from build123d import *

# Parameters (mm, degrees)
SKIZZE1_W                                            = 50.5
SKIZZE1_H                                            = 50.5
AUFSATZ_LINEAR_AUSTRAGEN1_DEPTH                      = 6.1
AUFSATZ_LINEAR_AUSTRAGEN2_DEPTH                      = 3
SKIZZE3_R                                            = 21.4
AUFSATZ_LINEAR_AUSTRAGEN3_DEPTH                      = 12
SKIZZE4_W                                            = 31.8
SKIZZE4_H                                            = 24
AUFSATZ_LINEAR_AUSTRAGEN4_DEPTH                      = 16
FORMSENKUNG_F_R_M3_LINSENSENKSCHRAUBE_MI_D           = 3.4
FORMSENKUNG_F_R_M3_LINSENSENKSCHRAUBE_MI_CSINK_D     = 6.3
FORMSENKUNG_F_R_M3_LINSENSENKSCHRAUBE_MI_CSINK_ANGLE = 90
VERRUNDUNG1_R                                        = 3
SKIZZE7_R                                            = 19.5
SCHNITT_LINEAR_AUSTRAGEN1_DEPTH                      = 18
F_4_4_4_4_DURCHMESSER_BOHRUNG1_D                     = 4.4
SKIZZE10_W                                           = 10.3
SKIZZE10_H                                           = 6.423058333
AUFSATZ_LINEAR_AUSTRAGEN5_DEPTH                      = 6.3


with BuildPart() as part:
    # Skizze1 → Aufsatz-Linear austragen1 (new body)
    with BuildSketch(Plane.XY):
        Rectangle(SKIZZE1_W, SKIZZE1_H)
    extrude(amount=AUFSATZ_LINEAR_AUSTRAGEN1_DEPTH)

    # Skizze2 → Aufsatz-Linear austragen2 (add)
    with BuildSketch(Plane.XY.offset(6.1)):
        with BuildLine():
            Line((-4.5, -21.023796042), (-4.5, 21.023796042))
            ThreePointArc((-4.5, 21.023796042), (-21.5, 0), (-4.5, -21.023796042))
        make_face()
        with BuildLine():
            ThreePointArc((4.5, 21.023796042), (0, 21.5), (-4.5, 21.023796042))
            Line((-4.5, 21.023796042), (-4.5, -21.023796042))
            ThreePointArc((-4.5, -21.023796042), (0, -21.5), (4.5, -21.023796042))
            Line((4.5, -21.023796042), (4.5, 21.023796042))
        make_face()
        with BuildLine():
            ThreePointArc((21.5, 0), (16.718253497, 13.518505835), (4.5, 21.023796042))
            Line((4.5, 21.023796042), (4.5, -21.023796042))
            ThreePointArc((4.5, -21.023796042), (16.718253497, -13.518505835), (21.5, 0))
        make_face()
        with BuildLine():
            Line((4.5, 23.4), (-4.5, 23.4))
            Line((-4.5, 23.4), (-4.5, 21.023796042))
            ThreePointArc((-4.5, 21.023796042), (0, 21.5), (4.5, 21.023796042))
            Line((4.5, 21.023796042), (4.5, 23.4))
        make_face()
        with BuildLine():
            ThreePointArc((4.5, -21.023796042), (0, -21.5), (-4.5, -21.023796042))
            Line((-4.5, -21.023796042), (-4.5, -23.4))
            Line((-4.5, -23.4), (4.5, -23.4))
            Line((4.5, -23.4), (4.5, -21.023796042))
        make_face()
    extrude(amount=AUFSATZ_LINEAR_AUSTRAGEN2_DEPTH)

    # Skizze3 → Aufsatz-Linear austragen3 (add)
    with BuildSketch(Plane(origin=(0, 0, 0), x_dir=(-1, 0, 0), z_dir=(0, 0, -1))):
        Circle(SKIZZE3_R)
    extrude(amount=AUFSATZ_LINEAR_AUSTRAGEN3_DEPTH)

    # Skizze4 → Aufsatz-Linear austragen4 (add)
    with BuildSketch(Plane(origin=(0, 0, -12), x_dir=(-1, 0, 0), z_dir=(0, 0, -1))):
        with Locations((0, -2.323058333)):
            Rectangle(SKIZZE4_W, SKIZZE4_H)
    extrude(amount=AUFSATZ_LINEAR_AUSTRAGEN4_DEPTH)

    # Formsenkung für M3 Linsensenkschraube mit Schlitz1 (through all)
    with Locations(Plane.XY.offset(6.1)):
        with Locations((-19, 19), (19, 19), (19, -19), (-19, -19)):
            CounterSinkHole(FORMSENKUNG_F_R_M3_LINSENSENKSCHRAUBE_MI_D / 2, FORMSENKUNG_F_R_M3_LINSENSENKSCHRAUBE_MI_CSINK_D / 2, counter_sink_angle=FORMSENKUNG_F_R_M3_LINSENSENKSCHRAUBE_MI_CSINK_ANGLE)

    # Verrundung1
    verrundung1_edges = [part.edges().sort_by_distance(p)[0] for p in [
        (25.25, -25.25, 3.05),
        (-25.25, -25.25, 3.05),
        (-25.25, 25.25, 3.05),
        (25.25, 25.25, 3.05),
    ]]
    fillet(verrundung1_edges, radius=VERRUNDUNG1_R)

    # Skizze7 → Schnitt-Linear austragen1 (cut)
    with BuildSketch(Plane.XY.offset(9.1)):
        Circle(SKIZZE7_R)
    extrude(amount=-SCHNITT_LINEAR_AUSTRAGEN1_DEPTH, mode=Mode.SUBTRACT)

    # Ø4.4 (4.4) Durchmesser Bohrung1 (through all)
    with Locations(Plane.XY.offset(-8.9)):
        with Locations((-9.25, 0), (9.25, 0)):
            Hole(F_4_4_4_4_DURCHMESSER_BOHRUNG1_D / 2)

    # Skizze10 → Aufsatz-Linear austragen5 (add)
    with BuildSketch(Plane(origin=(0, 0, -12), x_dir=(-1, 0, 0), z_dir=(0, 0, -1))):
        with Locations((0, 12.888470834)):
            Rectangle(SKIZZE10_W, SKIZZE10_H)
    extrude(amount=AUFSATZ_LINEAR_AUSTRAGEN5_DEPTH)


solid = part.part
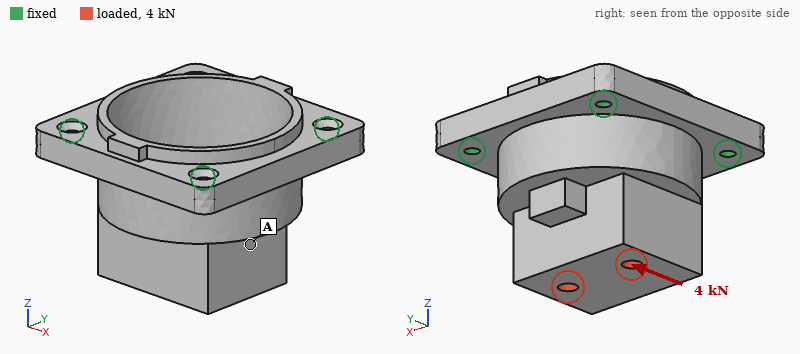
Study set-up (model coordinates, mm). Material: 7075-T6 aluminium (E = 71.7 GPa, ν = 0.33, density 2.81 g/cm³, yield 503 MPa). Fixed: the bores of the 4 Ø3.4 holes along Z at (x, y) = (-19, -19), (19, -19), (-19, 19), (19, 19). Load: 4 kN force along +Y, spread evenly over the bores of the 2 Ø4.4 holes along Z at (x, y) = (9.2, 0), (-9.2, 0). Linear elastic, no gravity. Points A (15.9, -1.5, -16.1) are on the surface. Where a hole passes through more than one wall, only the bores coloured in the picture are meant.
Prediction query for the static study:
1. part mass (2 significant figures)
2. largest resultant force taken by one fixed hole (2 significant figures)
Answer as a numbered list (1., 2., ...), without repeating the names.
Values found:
1. 77 g
2. 1.6 kN
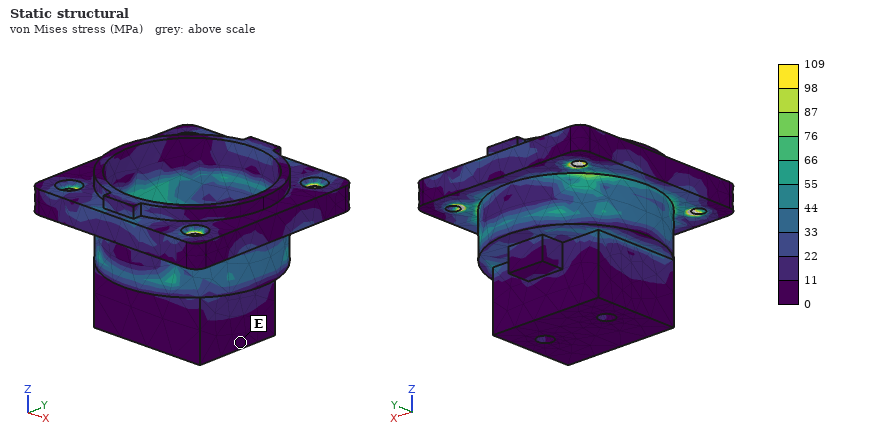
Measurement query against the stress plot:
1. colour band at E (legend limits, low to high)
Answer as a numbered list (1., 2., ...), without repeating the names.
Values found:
1. 0 to 11 MPa
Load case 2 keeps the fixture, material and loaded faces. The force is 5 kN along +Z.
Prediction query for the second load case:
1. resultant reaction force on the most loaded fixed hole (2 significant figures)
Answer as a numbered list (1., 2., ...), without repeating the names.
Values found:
1. 1.3 kN
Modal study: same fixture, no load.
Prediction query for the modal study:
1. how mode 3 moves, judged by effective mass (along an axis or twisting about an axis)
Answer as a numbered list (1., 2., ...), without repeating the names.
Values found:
1. along Z
